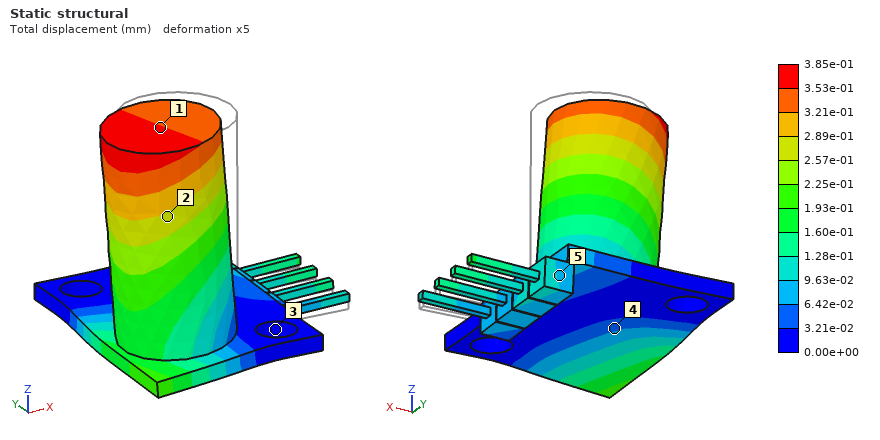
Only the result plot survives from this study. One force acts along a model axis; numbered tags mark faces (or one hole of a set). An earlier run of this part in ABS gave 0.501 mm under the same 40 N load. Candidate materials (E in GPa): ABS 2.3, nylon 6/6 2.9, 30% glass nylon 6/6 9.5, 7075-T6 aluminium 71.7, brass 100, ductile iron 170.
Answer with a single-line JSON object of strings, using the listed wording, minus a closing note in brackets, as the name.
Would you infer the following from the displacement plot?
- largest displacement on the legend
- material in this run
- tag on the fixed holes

{"largest displacement on the legend": "3.85e-01 mm", "material in this run": "nylon 6/6", "tag on the fixed holes": "3"}
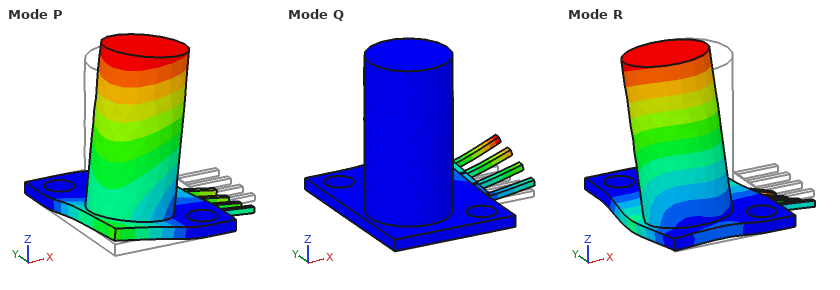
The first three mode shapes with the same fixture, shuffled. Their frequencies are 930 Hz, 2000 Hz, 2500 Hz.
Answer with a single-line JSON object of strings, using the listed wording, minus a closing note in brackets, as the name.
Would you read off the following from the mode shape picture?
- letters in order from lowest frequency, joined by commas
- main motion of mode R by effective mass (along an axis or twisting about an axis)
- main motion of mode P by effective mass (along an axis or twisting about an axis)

{"letters in order from lowest frequency, joined by commas": "P, R, Q", "main motion of mode R by effective mass": "along Y", "main motion of mode P by effective mass": "along X"}
